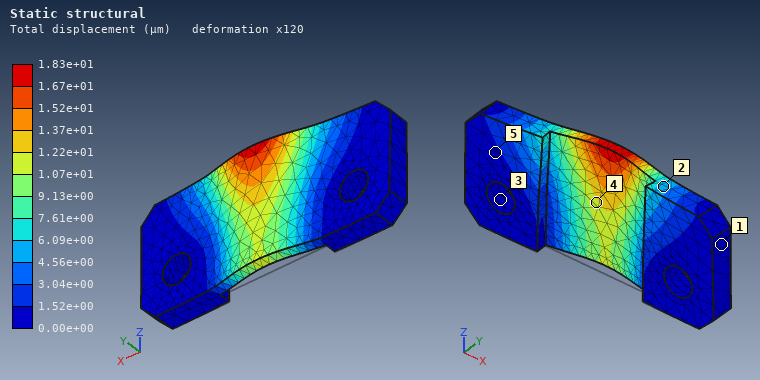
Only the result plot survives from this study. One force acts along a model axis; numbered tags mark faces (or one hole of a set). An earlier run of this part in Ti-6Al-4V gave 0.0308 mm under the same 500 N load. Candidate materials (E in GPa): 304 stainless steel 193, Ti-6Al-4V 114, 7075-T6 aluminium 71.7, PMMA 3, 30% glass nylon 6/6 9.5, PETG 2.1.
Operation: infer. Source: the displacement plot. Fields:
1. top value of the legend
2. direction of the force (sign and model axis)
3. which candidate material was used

1.83e+01 µm
+Y
304 stainless steel
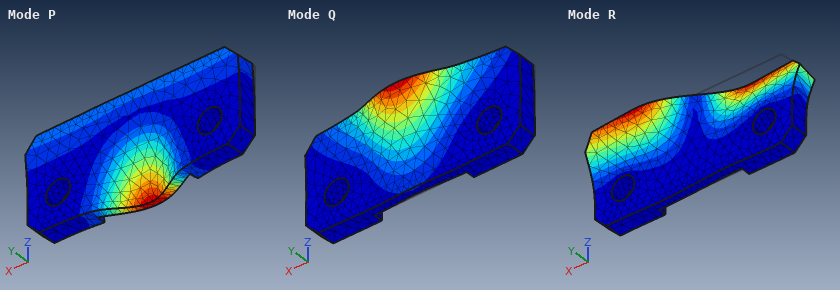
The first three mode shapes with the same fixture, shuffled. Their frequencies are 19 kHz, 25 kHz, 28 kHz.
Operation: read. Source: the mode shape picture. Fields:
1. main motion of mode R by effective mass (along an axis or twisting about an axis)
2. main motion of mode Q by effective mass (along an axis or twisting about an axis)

twisting about Z
along Y
